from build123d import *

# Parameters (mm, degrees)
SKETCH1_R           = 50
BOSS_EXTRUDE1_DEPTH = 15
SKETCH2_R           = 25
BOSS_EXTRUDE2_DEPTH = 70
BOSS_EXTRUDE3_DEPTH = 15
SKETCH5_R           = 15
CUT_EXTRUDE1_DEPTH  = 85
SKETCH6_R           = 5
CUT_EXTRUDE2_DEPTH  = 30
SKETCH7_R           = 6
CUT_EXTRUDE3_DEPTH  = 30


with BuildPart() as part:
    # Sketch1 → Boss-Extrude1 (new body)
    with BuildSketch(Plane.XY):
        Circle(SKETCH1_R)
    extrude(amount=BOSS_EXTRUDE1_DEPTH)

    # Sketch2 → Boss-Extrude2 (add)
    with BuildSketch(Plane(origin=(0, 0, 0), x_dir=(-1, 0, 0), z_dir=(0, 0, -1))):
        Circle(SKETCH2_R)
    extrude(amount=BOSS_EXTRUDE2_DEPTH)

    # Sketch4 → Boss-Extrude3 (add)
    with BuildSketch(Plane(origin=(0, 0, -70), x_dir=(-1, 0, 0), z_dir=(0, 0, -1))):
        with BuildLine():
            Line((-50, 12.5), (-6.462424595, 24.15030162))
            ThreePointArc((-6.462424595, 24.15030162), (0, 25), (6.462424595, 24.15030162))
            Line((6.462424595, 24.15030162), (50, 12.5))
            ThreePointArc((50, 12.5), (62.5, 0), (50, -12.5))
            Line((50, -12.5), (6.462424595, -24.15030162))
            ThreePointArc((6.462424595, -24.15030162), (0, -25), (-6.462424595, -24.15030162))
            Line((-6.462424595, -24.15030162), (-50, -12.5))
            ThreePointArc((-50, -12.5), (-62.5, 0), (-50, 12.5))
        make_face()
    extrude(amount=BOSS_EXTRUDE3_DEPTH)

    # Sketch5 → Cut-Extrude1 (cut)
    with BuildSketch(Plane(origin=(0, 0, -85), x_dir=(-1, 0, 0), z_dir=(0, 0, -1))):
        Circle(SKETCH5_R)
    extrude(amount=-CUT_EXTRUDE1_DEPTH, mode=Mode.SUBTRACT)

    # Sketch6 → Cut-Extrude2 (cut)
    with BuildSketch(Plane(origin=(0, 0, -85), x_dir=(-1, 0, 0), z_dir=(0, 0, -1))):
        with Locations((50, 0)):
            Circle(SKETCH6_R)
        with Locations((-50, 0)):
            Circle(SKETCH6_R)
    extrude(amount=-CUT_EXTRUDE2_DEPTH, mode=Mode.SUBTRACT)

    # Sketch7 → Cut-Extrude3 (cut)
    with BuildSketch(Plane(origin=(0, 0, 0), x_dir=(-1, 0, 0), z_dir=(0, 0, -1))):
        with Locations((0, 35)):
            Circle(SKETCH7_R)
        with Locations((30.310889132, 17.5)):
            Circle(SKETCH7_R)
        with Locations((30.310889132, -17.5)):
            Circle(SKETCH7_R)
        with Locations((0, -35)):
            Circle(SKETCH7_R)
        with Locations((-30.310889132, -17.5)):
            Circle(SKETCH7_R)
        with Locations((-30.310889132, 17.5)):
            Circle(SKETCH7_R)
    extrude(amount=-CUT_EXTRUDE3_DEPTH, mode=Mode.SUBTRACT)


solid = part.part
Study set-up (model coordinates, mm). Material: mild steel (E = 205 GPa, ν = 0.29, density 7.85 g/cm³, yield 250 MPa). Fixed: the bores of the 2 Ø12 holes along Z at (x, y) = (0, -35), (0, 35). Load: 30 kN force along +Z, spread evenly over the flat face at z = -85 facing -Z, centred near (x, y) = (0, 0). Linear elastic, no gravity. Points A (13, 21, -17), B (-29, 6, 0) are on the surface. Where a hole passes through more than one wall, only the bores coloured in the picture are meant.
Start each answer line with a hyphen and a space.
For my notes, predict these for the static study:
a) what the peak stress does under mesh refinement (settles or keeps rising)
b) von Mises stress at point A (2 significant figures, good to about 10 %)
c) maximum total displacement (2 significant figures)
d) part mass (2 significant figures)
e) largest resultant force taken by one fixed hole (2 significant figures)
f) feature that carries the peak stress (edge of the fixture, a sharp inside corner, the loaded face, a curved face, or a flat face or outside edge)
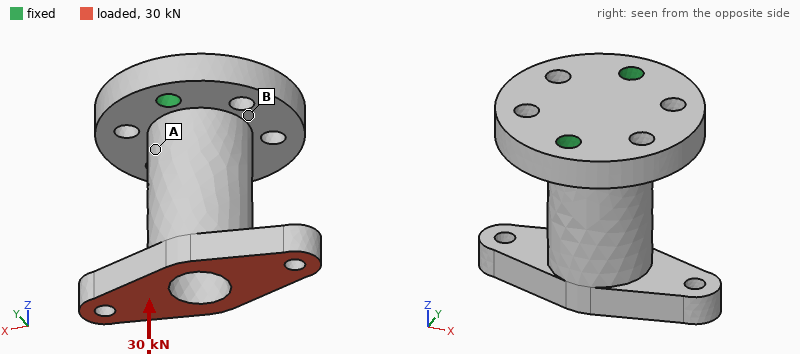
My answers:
- keeps rising
- 29 MPa
- 96 µm
- 1.9 kg
- 15 kN
- edge of the fixture
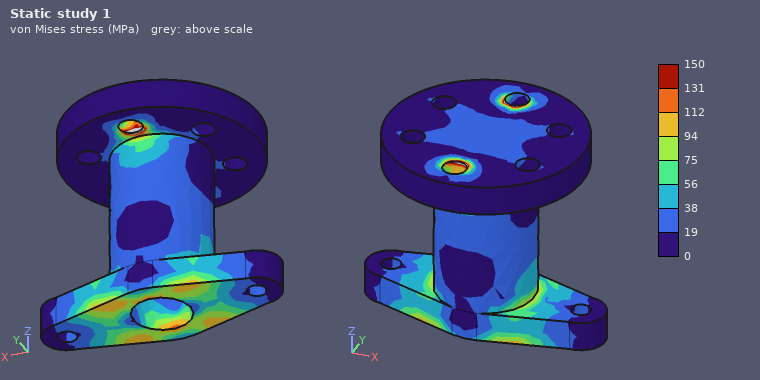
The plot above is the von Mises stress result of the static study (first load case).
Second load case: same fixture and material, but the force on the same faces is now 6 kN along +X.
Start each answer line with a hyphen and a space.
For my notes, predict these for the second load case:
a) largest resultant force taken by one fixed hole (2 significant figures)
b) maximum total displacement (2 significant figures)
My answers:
- 3.0 kN
- 0.16 mm
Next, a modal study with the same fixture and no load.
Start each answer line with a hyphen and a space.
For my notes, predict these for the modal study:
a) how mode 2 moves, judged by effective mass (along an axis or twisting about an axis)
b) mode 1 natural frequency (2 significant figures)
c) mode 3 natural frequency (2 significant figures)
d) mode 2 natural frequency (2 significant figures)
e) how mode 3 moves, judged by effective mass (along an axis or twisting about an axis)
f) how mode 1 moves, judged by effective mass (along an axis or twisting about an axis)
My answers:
- along Y
- 1400 Hz
- 4500 Hz
- 2600 Hz
- twisting about Z
- along X
